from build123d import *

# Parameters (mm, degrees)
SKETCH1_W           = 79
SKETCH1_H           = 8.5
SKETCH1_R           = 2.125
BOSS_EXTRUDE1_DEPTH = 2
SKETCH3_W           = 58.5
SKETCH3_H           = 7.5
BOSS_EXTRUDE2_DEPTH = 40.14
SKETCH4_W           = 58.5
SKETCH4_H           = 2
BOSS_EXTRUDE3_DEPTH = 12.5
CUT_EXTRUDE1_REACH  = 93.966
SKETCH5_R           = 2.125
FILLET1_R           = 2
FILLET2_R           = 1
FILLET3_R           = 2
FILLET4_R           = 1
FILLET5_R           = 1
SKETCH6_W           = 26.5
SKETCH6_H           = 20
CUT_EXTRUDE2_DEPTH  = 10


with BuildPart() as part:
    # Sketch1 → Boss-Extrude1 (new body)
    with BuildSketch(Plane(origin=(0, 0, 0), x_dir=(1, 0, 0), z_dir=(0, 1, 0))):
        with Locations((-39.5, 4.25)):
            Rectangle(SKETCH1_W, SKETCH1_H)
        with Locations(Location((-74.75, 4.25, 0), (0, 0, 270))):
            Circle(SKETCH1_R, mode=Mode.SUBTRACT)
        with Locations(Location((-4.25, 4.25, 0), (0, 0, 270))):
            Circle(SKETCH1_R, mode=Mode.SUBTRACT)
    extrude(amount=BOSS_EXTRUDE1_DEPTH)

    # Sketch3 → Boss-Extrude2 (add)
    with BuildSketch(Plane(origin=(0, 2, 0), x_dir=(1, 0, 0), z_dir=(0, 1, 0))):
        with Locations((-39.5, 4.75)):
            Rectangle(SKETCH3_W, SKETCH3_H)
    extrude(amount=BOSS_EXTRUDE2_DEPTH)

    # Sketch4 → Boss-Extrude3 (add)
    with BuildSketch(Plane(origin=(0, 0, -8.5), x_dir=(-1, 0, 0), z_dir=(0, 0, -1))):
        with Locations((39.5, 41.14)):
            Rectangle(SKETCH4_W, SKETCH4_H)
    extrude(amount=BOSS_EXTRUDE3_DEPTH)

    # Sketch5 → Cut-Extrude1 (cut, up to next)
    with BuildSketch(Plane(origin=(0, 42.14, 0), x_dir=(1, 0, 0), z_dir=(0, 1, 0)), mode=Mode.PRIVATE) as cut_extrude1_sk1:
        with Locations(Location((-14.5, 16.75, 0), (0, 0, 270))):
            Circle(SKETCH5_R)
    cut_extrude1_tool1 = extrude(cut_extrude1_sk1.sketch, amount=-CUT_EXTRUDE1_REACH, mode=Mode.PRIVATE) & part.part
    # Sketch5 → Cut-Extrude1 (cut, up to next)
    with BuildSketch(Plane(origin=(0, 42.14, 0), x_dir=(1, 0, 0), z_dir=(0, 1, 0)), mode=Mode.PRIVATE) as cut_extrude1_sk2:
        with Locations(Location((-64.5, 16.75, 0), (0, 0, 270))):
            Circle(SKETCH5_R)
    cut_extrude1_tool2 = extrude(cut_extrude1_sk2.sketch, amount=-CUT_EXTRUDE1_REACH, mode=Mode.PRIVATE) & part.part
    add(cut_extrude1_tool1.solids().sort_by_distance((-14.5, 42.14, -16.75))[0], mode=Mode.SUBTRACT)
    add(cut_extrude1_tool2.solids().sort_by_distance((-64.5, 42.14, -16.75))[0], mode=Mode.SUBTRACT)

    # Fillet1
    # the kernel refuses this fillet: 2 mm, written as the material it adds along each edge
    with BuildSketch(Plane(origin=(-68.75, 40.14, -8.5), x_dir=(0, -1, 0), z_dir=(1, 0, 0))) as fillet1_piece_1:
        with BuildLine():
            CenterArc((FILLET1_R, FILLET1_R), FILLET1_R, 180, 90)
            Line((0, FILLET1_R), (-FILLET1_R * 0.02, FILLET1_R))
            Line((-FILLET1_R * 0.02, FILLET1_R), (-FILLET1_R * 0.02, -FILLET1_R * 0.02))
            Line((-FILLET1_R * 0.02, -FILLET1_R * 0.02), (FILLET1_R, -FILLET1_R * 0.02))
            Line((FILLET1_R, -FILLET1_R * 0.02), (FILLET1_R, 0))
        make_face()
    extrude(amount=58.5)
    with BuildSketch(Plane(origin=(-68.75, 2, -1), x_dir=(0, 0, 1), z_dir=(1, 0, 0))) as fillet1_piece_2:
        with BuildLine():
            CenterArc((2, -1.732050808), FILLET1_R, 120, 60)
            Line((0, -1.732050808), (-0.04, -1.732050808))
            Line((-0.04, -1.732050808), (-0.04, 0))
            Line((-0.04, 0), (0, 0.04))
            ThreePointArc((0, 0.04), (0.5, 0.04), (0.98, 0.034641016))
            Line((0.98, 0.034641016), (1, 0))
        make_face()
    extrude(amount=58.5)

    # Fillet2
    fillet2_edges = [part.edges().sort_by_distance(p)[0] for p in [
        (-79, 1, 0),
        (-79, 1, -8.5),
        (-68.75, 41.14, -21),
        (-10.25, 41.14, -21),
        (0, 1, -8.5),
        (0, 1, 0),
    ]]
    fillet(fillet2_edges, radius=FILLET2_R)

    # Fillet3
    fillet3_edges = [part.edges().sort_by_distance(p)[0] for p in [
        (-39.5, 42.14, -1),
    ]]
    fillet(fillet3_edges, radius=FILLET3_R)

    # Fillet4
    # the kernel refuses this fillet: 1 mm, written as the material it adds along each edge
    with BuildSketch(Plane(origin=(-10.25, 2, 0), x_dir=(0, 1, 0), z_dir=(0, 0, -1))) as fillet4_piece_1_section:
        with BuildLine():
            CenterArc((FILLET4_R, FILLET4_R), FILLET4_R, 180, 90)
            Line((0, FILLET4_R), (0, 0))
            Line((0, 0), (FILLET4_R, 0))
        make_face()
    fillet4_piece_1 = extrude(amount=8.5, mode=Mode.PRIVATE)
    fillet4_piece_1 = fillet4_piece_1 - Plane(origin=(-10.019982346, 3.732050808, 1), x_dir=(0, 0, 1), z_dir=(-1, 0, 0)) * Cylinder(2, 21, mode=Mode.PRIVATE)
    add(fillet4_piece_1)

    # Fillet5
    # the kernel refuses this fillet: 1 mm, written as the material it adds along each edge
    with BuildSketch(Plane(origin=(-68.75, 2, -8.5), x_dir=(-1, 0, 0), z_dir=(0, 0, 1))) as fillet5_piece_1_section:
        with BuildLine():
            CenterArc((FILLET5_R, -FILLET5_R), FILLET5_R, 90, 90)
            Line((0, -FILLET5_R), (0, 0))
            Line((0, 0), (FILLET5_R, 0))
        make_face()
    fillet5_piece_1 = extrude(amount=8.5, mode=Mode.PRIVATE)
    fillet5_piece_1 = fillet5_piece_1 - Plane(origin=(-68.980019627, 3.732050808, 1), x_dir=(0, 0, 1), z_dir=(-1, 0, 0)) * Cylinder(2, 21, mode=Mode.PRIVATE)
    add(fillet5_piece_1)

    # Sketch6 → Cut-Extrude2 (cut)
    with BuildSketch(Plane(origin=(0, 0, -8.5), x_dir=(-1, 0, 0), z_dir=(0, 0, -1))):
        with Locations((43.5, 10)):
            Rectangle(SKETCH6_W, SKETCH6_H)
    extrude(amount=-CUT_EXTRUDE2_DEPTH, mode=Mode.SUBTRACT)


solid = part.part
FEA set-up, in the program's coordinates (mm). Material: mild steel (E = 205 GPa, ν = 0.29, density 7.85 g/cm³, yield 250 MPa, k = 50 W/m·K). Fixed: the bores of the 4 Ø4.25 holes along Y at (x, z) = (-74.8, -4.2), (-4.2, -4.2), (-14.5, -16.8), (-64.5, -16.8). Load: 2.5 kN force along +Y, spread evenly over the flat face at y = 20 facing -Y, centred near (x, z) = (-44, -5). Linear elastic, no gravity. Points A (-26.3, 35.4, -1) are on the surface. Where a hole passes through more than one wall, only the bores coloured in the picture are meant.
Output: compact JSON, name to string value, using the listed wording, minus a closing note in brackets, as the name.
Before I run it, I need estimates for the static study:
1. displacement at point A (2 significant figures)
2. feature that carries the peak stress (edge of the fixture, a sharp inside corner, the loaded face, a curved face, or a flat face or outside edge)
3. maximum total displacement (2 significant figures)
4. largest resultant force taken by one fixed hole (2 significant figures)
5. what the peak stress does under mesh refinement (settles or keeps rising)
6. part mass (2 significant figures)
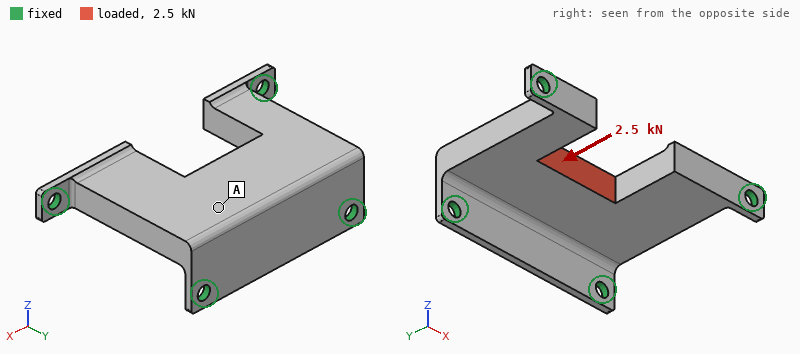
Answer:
{"displacement at point A": "15 µm", "feature that carries the peak stress": "edge of the fixture", "maximum total displacement": "18 µm", "largest resultant force taken by one fixed hole": "1.0 kN", "what the peak stress does under mesh refinement": "keeps rising", "part mass": "130 g"}
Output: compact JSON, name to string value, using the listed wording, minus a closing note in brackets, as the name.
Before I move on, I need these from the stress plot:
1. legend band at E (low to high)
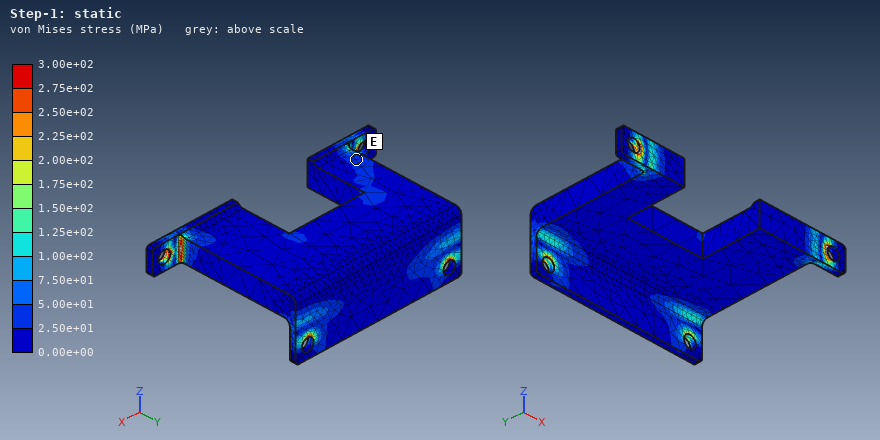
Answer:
{"legend band at E": "2.50e+01 to 5.00e+01 MPa"}
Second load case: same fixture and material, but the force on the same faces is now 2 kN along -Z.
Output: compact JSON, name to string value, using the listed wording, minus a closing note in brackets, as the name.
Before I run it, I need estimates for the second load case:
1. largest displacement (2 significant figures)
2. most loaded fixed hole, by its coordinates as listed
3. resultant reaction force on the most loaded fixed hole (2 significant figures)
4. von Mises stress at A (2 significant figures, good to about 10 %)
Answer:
{"largest displacement": "43 µm", "most loaded fixed hole, by its coordinates as listed": "(-64.5, -16.8)", "resultant reaction force on the most loaded fixed hole": "880 N", "von Mises stress at A": "41 MPa"}
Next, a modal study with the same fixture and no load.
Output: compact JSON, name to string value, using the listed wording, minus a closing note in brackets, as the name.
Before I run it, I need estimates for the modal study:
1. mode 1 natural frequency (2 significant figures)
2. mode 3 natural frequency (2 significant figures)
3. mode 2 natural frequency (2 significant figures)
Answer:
{"mode 1 natural frequency": "5600 Hz", "mode 3 natural frequency": "9700 Hz", "mode 2 natural frequency": "6800 Hz"}
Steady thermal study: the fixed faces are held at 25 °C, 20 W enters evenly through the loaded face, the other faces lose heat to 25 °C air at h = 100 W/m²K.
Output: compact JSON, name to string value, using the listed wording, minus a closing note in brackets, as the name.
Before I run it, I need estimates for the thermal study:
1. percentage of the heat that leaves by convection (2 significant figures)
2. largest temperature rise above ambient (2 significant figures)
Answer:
{"percentage of the heat that leaves by convection": "58 %", "largest temperature rise above ambient": "42 K"}
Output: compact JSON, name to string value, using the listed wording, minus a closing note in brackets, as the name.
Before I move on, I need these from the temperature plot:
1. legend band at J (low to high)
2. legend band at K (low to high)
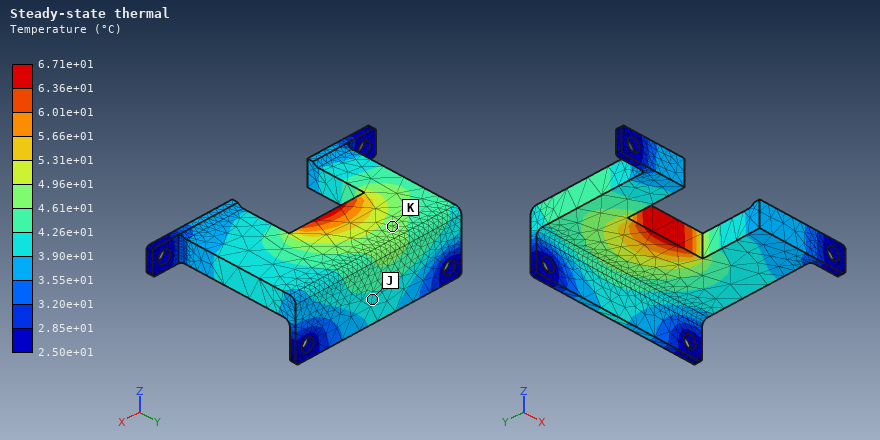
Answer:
{"legend band at J": "3.90e+01 to 4.26e+01 °C", "legend band at K": "4.61e+01 to 4.96e+01 °C"}
